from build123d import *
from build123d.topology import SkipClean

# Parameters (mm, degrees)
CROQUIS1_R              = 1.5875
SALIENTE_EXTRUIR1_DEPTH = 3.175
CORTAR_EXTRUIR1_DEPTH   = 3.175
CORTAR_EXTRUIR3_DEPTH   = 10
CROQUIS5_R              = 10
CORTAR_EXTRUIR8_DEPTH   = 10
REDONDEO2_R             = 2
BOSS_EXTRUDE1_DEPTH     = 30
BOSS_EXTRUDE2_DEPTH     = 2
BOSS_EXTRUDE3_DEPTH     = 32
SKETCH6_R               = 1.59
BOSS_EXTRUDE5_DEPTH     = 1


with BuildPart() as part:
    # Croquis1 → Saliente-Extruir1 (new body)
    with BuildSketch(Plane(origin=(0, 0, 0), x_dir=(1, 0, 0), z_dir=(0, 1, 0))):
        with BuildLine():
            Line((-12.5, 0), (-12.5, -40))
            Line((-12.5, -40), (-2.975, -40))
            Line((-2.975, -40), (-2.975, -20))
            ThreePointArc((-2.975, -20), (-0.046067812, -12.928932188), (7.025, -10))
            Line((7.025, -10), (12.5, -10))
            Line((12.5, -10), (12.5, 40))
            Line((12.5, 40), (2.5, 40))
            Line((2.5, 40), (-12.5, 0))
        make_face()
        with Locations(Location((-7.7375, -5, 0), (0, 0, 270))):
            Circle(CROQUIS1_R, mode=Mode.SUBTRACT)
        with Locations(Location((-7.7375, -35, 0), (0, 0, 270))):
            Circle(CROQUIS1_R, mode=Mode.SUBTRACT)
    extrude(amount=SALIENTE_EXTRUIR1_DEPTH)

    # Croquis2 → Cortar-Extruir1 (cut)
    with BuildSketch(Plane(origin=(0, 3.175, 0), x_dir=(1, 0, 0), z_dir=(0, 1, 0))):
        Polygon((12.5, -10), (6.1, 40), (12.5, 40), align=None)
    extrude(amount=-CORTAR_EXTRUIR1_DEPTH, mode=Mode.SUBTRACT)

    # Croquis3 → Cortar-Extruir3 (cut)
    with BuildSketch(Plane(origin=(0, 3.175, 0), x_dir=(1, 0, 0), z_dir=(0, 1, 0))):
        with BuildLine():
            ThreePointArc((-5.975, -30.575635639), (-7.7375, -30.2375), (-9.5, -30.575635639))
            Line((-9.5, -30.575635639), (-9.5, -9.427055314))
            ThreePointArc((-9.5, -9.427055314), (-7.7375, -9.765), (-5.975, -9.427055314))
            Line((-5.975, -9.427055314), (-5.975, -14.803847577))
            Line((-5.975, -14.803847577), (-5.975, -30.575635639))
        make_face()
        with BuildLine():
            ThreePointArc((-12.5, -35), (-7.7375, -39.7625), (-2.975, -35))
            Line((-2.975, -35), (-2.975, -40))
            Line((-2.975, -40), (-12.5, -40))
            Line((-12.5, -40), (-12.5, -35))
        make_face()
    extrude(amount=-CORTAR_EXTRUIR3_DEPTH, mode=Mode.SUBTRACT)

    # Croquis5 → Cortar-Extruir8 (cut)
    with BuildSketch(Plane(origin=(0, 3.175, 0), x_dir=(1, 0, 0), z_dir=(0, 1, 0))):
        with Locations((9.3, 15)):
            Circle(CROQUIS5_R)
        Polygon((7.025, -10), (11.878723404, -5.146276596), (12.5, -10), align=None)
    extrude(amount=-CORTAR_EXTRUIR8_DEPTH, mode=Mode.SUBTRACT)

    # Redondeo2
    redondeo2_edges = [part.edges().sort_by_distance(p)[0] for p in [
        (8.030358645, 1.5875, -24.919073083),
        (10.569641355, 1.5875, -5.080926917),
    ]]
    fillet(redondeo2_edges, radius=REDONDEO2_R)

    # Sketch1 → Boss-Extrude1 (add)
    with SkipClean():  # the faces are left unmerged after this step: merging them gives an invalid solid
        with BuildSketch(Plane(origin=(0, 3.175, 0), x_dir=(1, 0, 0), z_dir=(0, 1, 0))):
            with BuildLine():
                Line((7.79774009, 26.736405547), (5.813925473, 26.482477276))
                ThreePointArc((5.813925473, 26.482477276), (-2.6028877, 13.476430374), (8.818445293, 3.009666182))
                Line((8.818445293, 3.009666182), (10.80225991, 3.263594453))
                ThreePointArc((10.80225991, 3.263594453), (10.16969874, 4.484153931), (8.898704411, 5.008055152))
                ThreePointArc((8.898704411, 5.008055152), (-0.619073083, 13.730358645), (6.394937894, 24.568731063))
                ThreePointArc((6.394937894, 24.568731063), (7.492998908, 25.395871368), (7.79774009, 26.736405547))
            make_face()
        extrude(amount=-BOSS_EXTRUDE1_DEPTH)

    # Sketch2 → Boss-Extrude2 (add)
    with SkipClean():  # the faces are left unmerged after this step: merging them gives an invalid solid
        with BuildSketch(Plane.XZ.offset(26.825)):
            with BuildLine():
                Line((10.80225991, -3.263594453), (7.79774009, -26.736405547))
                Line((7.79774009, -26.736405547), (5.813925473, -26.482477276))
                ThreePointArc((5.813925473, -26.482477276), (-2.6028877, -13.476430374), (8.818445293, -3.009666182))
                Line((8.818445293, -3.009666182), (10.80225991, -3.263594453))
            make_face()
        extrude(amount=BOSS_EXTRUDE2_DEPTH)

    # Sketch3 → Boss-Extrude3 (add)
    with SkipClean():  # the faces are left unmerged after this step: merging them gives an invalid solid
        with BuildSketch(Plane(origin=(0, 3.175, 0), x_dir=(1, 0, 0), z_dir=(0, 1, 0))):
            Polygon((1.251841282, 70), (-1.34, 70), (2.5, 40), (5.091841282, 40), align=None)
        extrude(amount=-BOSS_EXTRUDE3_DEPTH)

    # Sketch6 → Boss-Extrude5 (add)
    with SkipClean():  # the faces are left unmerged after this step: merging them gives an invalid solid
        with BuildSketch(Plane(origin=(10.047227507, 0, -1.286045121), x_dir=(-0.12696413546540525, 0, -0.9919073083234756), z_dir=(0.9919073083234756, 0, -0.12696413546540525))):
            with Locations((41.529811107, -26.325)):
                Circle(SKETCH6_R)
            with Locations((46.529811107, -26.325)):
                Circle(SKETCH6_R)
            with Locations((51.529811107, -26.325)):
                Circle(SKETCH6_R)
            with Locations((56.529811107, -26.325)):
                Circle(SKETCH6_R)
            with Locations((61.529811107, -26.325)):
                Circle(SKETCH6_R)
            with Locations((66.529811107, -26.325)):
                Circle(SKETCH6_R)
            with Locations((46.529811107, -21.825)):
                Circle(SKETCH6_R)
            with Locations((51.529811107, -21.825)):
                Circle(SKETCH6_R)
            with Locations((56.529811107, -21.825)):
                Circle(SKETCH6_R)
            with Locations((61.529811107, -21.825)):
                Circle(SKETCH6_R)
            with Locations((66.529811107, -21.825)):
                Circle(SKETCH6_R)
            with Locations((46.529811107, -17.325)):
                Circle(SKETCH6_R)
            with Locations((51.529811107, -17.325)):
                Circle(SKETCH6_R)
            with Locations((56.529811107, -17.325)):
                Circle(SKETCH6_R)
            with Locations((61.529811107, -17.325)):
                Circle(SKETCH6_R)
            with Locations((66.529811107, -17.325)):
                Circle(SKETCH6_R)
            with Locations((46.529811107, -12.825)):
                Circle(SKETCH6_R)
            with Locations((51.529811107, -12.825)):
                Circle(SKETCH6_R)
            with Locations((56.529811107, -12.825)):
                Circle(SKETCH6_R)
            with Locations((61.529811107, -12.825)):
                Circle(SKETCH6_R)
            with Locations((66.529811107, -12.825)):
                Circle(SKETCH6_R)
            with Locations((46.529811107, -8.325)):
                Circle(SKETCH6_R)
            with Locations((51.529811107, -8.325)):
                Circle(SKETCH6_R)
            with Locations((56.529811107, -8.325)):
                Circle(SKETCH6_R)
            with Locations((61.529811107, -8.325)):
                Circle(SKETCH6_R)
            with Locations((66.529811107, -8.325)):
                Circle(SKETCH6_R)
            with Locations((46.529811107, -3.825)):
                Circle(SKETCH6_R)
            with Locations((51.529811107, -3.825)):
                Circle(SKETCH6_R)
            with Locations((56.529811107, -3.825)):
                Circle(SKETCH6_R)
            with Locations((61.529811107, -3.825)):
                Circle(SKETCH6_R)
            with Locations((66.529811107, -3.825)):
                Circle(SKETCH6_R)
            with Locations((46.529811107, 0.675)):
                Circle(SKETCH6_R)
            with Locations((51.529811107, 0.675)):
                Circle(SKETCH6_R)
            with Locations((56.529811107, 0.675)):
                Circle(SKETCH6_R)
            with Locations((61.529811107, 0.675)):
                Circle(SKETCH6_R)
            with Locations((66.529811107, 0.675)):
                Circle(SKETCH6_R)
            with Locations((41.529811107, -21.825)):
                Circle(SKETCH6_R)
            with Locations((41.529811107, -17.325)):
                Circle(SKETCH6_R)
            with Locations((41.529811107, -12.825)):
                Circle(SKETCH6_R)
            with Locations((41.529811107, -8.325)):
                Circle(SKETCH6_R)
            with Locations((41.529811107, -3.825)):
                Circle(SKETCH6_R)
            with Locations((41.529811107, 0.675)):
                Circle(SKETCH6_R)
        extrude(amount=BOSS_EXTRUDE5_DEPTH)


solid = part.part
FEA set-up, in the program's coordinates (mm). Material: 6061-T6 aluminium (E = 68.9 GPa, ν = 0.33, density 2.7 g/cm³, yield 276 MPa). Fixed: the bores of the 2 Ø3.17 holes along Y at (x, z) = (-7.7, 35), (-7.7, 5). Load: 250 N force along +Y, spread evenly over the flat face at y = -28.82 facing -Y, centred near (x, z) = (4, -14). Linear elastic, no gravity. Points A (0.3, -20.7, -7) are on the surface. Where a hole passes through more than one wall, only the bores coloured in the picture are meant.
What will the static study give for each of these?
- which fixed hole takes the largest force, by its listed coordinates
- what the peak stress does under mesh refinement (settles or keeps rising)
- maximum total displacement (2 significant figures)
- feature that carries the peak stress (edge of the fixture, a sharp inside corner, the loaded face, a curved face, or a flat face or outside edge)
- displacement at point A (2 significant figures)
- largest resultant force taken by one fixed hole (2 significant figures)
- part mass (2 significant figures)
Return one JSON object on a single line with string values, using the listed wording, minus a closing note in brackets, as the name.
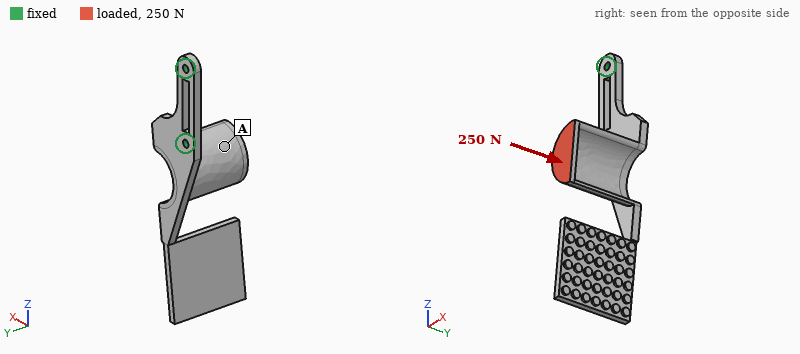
{"which fixed hole takes the largest force, by its listed coordinates": "(-7.7, 5)", "what the peak stress does under mesh refinement": "keeps rising", "maximum total displacement": "1.4 mm", "feature that carries the peak stress": "edge of the fixture", "displacement at point A": "0.45 mm", "largest resultant force taken by one fixed hole": "280 N", "part mass": "21 g"}
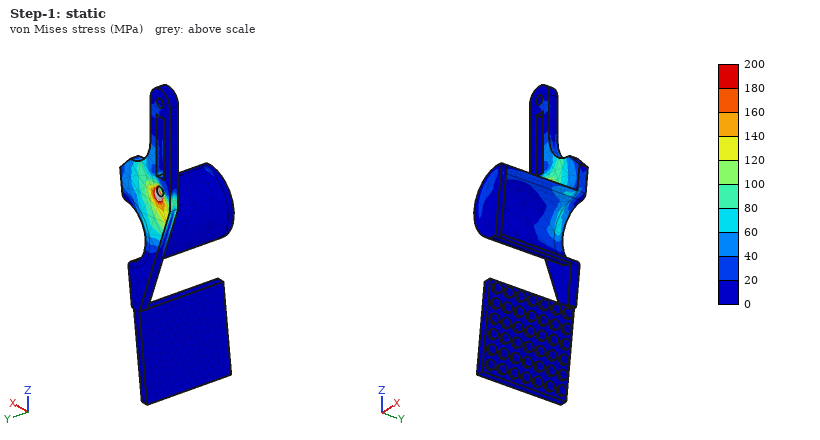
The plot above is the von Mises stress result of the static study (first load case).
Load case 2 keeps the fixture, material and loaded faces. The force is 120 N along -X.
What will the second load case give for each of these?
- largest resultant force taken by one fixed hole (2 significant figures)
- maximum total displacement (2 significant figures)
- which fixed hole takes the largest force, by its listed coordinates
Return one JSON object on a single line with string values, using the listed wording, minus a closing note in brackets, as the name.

{"largest resultant force taken by one fixed hole": "150 N", "maximum total displacement": "0.76 mm", "which fixed hole takes the largest force, by its listed coordinates": "(-7.7, 5)"}
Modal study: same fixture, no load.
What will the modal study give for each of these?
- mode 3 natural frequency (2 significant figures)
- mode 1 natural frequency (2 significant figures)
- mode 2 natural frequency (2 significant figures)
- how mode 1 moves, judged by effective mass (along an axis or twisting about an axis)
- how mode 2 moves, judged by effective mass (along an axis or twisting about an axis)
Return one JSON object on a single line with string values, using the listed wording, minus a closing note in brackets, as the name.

{"mode 3 natural frequency": "1000 Hz", "mode 1 natural frequency": "310 Hz", "mode 2 natural frequency": "430 Hz", "how mode 1 moves, judged by effective mass": "along Y", "how mode 2 moves, judged by effective mass": "along X"}
